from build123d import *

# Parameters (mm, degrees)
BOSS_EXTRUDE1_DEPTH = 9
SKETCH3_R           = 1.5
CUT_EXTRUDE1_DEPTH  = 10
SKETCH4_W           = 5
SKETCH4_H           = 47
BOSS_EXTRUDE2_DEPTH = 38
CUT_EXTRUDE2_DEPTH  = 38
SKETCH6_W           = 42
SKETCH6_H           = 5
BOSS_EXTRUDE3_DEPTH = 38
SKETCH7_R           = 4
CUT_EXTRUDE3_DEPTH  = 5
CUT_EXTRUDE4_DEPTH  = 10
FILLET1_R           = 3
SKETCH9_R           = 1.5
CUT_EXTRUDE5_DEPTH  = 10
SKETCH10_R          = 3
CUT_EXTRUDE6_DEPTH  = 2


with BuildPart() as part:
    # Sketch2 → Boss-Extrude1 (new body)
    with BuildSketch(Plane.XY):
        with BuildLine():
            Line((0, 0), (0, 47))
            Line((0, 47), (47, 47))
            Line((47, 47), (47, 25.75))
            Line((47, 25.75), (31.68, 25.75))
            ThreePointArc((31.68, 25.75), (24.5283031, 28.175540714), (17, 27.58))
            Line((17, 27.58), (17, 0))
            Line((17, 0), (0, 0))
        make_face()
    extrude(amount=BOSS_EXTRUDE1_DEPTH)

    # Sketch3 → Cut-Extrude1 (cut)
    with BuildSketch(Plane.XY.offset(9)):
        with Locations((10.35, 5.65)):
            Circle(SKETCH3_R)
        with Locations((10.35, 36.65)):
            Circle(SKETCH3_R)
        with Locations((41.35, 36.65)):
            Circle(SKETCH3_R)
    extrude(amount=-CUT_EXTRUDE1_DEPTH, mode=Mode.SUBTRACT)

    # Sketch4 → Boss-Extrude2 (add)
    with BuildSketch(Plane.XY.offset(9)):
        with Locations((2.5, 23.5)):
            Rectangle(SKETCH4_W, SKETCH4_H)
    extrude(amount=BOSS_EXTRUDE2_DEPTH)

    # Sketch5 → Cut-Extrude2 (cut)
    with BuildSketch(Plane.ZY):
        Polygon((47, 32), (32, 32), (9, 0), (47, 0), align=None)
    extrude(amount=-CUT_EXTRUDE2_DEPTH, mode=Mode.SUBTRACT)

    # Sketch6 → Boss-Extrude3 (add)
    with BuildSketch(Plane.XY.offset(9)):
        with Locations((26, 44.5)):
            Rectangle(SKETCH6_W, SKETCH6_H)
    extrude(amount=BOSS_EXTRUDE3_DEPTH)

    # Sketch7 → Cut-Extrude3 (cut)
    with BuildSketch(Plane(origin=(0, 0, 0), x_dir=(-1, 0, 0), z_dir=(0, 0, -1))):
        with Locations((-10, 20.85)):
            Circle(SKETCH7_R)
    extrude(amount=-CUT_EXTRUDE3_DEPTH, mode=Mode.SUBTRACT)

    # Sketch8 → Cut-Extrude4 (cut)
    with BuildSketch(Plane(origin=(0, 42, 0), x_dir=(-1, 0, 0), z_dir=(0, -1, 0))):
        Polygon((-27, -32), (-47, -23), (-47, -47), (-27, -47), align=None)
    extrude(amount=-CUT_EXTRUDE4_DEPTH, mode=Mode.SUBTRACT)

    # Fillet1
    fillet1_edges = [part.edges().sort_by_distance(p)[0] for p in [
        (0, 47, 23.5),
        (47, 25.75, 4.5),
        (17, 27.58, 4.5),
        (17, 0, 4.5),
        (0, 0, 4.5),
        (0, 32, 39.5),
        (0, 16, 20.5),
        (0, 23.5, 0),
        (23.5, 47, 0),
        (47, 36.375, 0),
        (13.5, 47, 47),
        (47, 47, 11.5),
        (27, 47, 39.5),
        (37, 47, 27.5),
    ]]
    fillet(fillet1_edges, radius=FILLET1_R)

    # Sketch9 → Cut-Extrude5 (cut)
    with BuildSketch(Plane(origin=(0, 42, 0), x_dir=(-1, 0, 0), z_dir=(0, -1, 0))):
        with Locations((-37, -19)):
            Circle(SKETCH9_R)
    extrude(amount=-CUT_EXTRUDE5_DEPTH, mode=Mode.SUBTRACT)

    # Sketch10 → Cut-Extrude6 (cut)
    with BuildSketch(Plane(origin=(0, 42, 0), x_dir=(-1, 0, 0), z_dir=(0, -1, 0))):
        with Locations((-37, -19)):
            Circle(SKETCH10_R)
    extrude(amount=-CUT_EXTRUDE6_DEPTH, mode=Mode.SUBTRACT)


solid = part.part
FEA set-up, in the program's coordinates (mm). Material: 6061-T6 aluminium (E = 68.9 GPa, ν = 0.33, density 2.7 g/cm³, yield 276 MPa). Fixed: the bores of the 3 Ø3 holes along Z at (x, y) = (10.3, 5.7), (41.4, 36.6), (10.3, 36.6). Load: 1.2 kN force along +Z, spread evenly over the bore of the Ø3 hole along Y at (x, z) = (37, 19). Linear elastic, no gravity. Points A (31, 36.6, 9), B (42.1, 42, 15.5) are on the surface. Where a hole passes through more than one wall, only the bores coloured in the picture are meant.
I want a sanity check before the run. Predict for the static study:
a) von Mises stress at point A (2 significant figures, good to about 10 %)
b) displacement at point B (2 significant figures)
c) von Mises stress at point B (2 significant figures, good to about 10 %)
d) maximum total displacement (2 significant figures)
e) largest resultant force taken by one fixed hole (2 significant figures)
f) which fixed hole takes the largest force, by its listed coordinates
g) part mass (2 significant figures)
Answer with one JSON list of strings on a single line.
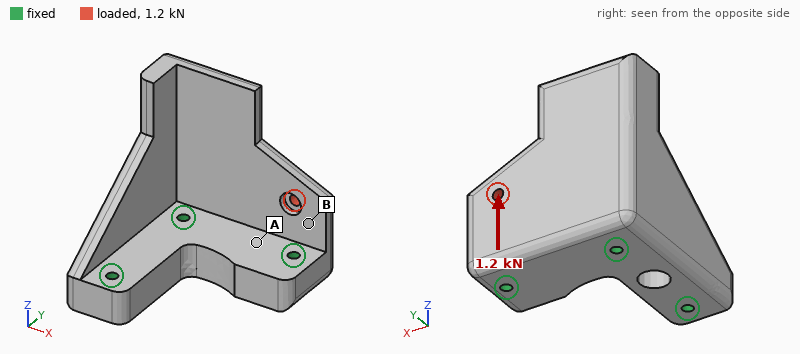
["7.1 MPa", "11 µm", "15 MPa", "22 µm", "990 N", "(41.4, 36.6)", "60 g"]
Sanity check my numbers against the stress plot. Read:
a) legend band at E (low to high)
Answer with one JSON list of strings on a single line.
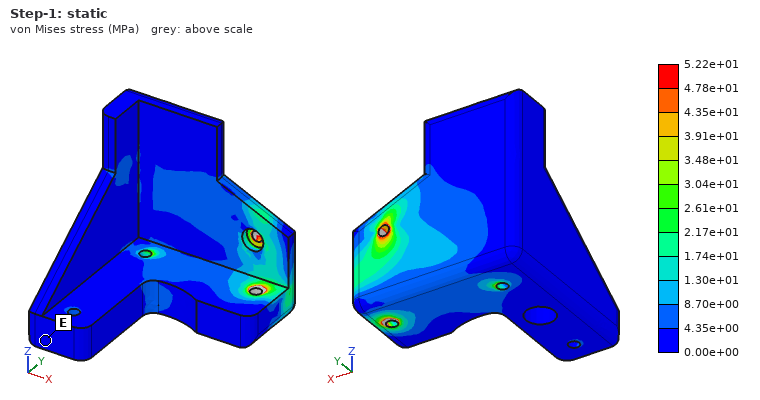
["0.00e+00 to 4.35e+00 MPa"]
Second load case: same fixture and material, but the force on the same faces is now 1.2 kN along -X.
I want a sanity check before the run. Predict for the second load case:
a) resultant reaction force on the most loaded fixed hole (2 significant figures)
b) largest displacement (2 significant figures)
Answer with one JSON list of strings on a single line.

["850 N", "11 µm"]
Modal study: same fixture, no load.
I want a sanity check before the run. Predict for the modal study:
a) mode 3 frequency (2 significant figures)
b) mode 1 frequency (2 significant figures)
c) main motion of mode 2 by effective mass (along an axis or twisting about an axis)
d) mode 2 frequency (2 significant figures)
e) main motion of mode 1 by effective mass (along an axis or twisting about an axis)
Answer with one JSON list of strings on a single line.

["13 kHz", "5800 Hz", "along X", "8300 Hz", "along Y"]
